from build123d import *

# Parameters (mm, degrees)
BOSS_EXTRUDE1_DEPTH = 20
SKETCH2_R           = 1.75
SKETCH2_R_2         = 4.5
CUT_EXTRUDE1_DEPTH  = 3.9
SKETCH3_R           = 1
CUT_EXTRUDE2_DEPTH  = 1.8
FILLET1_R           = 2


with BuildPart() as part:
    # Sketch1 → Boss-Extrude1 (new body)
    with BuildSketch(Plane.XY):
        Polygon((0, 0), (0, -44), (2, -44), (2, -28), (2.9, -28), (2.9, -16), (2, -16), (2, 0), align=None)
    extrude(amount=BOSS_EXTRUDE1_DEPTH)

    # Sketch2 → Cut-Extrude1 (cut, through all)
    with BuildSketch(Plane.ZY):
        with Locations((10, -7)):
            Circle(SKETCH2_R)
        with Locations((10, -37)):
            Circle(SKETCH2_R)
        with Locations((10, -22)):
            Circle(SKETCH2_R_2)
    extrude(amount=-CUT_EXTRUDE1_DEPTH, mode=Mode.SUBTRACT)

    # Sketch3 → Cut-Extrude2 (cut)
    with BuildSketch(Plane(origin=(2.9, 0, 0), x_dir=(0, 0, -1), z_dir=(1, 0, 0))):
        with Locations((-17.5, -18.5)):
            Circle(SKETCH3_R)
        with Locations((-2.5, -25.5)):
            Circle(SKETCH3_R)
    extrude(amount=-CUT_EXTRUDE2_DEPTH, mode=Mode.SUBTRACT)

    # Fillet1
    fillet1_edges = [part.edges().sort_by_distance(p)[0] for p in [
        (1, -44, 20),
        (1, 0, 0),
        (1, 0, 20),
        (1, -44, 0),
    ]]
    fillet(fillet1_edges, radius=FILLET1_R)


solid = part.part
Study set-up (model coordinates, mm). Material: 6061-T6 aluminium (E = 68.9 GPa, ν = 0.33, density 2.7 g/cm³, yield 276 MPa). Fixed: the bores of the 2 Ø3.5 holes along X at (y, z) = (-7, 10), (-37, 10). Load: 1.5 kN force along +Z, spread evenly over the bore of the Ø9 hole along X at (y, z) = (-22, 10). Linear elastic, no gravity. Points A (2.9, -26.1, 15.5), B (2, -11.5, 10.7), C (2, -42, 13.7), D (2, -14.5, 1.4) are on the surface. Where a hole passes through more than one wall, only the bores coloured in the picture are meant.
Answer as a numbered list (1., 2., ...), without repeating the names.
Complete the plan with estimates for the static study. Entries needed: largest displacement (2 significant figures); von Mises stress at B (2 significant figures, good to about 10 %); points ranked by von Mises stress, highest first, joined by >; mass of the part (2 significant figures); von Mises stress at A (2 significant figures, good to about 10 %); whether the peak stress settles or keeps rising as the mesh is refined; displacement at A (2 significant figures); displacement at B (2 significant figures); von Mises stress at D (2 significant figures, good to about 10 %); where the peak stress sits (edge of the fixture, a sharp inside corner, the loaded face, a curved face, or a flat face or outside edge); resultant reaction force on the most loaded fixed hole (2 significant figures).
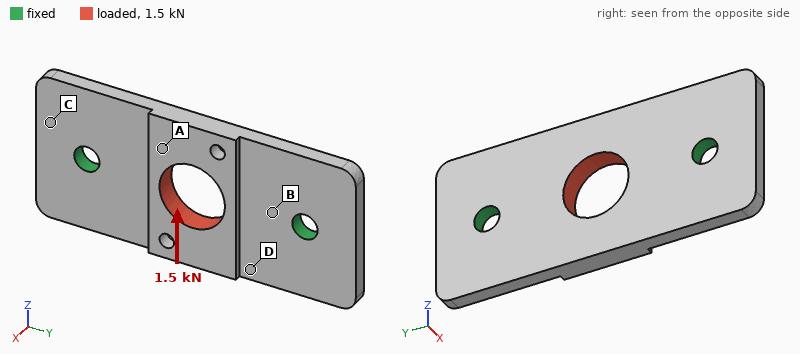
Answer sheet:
1. 32 µm
2. 68 MPa
3. B > D > A > C
4. 4.7 g
5. 26 MPa
6. keeps rising
7. 22 µm
8. 6.9 µm
9. 38 MPa
10. edge of the fixture
11. 750 N
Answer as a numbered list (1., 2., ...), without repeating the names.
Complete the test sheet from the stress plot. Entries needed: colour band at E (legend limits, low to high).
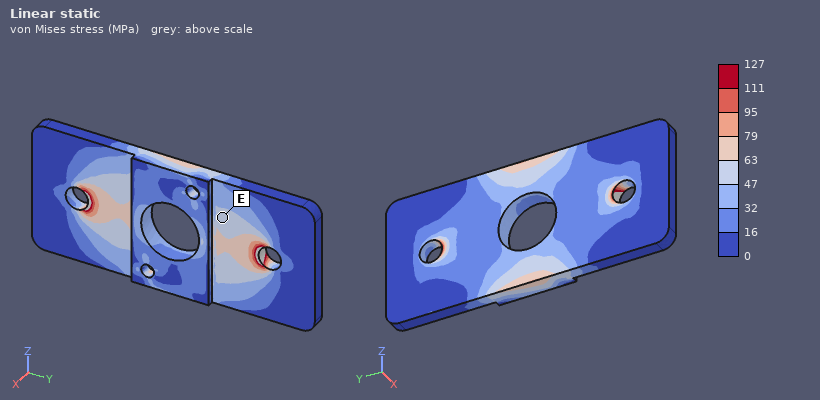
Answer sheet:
1. 47 to 63 MPa
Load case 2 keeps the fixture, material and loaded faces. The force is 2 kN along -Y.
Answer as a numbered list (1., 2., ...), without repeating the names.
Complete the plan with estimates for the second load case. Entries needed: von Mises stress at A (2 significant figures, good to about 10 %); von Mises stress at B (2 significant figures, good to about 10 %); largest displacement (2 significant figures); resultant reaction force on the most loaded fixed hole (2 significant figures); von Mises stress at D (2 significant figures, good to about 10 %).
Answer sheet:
1. 14 MPa
2. 61 MPa
3. 8.4 µm
4. 1.0 kN
5. 15 MPa
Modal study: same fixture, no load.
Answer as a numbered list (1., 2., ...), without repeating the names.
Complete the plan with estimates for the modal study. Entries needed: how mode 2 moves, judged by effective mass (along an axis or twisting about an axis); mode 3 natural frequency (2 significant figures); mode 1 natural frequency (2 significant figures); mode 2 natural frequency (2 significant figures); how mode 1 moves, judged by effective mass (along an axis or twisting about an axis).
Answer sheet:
1. along X
2. 19 kHz
3. 10 kHz
4. 11 kHz
5. twisting about Y
